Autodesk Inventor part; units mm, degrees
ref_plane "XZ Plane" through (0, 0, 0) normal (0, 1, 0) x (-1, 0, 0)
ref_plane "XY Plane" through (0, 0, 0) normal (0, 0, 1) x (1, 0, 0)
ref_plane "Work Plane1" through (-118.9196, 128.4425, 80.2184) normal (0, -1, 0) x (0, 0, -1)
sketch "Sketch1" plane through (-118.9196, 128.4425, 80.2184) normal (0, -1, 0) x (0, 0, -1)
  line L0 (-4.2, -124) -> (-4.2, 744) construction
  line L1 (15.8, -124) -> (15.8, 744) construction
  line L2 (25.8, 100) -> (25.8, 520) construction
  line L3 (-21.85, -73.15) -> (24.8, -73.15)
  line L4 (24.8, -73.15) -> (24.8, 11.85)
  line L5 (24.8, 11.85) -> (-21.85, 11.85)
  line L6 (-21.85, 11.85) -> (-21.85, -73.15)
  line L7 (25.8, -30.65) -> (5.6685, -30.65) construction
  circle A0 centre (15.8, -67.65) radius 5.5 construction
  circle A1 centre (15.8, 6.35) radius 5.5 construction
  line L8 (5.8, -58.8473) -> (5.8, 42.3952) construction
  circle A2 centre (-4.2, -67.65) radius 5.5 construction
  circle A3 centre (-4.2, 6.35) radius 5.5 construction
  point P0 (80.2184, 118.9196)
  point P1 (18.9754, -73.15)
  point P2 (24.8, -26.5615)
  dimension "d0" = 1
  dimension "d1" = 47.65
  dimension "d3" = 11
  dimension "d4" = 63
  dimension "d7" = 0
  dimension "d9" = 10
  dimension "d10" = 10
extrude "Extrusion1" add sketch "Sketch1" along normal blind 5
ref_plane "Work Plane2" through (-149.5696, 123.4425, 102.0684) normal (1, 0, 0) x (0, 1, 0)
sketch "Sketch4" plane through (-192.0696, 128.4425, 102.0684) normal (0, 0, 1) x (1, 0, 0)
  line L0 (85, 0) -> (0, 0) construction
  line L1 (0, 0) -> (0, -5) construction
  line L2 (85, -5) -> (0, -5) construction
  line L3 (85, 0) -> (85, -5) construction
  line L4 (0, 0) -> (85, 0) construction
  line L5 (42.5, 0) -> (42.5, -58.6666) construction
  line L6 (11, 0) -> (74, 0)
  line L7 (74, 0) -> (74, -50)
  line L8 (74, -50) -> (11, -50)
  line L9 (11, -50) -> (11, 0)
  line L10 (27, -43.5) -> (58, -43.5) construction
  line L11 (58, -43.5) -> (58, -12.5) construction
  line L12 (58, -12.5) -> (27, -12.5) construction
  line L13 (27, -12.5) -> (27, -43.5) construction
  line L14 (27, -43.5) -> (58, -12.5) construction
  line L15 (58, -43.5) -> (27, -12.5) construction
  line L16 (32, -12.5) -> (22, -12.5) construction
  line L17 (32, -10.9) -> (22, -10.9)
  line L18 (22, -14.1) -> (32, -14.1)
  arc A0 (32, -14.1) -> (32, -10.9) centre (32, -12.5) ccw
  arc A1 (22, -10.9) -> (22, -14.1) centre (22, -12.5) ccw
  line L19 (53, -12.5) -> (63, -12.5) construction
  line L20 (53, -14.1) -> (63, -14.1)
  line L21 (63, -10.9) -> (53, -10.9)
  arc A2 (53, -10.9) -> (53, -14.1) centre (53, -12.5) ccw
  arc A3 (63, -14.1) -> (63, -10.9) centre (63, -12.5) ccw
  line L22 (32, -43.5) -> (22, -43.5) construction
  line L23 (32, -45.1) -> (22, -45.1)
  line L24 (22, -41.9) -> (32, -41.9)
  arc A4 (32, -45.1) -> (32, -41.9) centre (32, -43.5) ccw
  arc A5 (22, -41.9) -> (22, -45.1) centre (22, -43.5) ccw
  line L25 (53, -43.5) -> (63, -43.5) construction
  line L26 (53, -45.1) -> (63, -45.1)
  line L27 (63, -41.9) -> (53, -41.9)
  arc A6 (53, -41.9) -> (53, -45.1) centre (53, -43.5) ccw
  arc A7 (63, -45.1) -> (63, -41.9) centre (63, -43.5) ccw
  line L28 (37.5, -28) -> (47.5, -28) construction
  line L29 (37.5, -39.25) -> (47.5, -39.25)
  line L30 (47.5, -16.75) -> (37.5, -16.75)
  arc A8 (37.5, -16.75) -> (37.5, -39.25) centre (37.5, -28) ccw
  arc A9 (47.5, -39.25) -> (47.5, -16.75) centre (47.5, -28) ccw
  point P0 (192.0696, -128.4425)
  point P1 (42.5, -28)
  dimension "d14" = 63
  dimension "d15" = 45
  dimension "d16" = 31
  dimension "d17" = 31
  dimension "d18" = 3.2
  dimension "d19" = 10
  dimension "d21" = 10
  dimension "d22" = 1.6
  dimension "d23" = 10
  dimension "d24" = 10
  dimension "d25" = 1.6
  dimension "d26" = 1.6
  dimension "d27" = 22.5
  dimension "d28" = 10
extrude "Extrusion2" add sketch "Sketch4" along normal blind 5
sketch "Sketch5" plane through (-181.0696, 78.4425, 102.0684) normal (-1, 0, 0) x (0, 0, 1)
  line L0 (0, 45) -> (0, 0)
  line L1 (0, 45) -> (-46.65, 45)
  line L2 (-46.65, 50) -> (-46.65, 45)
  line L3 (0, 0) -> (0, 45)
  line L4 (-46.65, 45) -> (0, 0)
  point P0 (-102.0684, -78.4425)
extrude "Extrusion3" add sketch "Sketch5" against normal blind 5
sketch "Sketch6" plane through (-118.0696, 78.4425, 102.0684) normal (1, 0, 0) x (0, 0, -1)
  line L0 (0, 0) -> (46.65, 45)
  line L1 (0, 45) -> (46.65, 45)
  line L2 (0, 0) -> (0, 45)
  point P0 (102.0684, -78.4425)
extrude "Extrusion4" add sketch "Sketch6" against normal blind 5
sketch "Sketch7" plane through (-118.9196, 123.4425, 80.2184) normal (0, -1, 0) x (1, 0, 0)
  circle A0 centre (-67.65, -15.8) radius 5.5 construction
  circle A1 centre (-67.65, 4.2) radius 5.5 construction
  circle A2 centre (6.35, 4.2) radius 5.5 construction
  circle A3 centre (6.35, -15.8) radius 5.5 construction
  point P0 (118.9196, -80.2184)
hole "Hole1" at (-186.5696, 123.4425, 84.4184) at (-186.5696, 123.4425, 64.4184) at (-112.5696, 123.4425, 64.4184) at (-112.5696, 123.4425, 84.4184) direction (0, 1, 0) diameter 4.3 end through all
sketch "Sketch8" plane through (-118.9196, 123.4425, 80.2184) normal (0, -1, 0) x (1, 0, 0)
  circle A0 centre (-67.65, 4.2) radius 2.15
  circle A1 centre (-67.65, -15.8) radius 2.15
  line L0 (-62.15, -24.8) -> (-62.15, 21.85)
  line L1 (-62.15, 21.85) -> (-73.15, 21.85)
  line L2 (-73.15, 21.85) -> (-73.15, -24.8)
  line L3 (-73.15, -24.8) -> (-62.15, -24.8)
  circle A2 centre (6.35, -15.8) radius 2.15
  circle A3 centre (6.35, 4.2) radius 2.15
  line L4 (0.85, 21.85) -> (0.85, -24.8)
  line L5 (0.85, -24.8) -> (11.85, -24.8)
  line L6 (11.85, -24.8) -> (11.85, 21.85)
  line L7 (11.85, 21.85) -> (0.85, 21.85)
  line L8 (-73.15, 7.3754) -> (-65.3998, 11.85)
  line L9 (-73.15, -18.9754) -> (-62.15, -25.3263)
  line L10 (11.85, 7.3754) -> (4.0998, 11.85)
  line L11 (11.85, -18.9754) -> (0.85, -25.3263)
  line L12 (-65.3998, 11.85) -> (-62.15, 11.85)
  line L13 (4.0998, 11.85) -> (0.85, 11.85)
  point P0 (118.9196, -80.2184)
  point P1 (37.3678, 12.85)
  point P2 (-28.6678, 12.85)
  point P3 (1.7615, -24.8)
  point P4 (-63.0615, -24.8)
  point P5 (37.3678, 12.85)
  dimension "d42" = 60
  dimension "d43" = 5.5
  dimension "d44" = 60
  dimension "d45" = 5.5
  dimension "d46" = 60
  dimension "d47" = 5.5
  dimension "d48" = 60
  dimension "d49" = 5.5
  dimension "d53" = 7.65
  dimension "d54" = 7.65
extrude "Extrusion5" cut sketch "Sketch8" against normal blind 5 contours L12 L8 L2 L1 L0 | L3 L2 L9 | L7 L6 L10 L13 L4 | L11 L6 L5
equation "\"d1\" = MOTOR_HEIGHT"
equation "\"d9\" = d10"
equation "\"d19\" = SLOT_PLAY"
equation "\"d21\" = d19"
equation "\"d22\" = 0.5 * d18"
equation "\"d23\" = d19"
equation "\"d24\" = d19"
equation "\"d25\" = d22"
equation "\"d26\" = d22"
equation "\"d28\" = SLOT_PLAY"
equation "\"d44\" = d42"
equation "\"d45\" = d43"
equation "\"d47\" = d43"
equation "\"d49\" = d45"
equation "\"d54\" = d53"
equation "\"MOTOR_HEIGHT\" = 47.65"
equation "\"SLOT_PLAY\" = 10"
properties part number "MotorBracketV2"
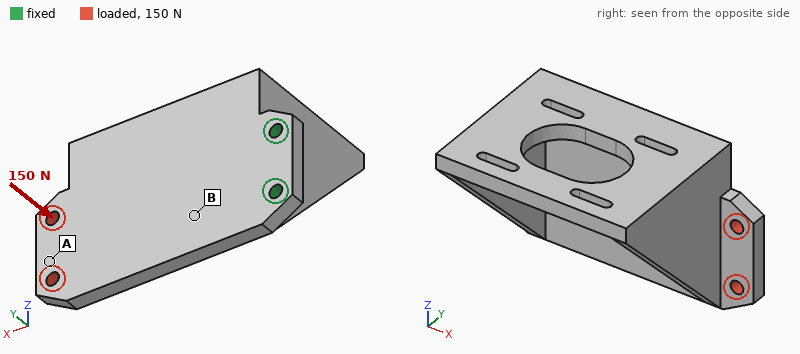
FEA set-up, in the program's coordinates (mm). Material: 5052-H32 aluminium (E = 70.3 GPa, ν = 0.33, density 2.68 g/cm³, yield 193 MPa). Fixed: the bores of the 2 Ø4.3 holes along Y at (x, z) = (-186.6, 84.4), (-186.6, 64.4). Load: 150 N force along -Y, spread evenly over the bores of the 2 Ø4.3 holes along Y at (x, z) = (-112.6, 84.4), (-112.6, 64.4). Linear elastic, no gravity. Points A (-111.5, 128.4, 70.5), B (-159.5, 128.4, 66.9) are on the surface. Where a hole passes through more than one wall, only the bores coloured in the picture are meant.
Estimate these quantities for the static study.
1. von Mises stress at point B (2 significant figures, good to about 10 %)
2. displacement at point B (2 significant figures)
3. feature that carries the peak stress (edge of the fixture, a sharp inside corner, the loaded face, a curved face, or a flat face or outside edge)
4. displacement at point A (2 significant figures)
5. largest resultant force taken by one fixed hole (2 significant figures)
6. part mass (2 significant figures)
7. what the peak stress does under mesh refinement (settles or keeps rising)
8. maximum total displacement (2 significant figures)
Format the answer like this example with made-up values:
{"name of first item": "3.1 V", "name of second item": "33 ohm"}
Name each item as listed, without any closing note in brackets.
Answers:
{"von Mises stress at point B": "16 MPa", "displacement at point B": "0.091 mm", "feature that carries the peak stress": "edge of the fixture", "displacement at point A": "0.39 mm", "largest resultant force taken by one fixed hole": "84 N", "part mass": "110 g", "what the peak stress does under mesh refinement": "keeps rising", "maximum total displacement": "0.42 mm"}
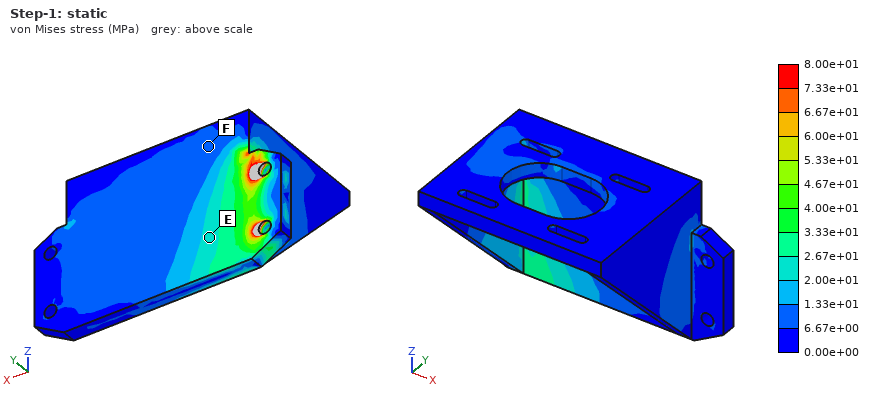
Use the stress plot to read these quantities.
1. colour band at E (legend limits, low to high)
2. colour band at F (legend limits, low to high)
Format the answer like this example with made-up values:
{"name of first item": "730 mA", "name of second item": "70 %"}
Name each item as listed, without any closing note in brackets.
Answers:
{"colour band at E": "2.00e+01 to 2.67e+01 MPa", "colour band at F": "6.67e+00 to 1.33e+01 MPa"}
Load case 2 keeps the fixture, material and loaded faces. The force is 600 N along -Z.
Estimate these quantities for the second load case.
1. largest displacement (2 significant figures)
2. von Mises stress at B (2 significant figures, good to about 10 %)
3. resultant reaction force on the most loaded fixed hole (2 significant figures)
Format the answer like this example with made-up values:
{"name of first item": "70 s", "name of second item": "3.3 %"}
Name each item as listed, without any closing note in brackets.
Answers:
{"largest displacement": "69 µm", "von Mises stress at B": "11 MPa", "resultant reaction force on the most loaded fixed hole": "2.0 kN"}
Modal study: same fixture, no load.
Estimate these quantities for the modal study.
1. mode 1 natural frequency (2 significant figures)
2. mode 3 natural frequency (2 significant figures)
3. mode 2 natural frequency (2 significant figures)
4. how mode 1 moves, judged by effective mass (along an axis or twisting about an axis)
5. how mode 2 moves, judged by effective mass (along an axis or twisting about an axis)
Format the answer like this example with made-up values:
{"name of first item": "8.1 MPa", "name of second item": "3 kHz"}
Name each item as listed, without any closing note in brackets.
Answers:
{"mode 1 natural frequency": "500 Hz", "mode 3 natural frequency": "2700 Hz", "mode 2 natural frequency": "1400 Hz", "how mode 1 moves, judged by effective mass": "along Y", "how mode 2 moves, judged by effective mass": "along Z"}
